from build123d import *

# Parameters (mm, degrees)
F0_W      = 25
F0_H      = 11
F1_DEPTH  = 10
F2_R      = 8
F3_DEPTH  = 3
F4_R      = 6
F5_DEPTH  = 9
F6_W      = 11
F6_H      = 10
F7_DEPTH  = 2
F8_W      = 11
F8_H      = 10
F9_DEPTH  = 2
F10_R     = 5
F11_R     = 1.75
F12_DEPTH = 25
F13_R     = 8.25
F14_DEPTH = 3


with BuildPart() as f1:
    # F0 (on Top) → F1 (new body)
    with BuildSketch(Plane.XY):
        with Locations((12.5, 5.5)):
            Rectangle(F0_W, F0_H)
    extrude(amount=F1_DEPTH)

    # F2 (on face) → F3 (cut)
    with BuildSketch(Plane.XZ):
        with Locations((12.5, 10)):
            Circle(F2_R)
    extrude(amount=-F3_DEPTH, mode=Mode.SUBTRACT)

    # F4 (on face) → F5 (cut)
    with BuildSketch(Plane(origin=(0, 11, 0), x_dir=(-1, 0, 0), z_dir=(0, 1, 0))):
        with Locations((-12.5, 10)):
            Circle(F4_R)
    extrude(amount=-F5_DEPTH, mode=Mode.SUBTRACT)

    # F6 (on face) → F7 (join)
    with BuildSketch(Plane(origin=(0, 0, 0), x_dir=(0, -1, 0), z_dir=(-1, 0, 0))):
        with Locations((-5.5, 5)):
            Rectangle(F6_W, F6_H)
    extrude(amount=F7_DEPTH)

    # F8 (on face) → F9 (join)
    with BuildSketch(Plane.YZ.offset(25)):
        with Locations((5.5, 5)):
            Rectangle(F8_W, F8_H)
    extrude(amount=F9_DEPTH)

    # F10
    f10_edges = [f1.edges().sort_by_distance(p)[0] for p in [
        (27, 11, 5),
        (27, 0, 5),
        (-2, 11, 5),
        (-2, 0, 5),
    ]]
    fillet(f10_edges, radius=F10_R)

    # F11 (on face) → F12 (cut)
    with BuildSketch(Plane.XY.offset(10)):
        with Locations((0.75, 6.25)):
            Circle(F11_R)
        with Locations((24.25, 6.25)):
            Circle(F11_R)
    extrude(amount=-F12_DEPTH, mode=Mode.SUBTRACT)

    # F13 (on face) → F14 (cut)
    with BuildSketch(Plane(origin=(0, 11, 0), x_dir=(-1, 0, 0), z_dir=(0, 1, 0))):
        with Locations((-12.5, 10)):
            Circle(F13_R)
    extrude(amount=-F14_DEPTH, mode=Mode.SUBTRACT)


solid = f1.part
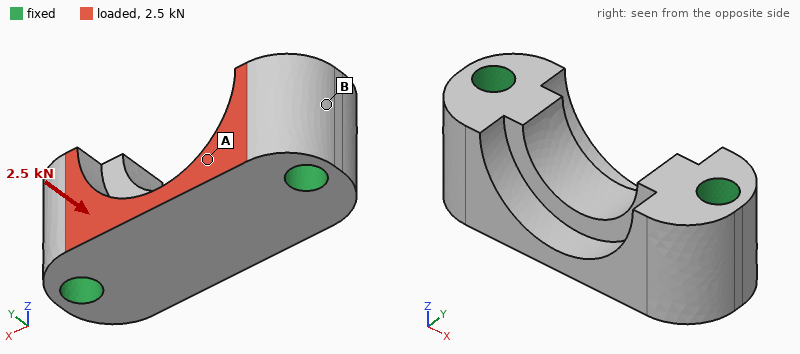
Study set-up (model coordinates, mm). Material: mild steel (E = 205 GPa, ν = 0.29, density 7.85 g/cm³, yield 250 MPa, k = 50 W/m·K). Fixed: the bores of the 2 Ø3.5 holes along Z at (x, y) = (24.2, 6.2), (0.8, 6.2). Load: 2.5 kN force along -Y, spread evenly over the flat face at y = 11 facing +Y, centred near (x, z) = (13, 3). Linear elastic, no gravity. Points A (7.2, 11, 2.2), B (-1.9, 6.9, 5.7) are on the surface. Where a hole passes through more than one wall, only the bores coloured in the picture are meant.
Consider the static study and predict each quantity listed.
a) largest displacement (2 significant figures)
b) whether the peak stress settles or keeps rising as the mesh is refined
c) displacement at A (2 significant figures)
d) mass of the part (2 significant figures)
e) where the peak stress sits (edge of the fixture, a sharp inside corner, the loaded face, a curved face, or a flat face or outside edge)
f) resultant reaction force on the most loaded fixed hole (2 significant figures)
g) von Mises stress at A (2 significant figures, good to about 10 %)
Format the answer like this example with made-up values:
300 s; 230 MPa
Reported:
4.2 µm; keeps rising; 2.8 µm; 15 g; edge of the fixture; 1.3 kN; 31 MPa
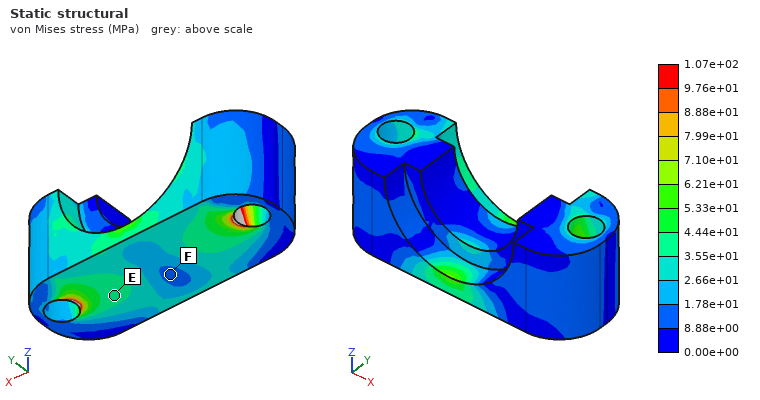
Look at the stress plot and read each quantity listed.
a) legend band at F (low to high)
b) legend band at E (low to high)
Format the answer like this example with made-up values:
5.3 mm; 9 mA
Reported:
8.88e+00 to 1.78e+01 MPa; 3.55e+01 to 4.44e+01 MPa
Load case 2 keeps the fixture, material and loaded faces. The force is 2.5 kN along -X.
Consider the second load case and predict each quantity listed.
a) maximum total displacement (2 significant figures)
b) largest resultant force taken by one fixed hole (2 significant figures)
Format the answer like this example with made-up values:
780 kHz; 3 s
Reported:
2.0 µm; 1.3 kN
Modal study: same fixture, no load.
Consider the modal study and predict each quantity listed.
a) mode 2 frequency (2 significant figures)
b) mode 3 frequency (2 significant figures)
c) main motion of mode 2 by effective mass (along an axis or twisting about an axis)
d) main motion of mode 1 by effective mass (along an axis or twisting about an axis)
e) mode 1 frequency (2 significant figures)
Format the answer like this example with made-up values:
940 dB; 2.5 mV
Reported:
66 kHz; 87 kHz; along Z; along Y; 53 kHz
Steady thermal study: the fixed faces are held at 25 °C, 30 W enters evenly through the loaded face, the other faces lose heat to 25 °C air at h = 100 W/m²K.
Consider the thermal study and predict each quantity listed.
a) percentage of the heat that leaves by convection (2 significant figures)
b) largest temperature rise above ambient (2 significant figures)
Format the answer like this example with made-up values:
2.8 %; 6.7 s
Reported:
3.3 %; 45 K
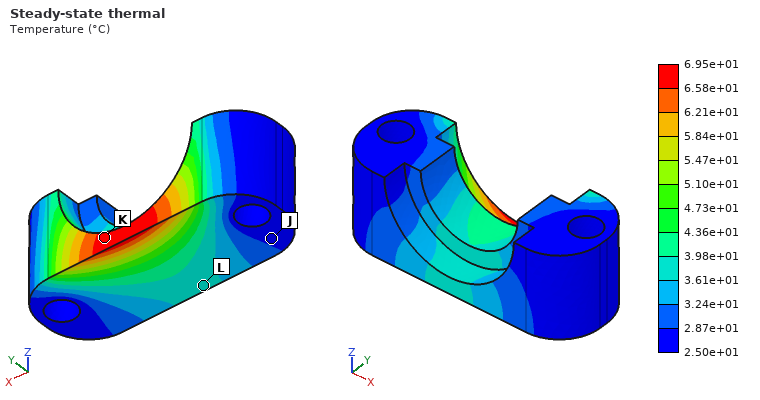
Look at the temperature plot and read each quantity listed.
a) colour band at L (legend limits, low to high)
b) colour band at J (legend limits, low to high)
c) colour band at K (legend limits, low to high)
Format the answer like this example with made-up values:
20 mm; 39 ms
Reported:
3.61e+01 to 3.98e+01 °C; 2.50e+01 to 2.87e+01 °C; 6.58e+01 to 6.95e+01 °C
